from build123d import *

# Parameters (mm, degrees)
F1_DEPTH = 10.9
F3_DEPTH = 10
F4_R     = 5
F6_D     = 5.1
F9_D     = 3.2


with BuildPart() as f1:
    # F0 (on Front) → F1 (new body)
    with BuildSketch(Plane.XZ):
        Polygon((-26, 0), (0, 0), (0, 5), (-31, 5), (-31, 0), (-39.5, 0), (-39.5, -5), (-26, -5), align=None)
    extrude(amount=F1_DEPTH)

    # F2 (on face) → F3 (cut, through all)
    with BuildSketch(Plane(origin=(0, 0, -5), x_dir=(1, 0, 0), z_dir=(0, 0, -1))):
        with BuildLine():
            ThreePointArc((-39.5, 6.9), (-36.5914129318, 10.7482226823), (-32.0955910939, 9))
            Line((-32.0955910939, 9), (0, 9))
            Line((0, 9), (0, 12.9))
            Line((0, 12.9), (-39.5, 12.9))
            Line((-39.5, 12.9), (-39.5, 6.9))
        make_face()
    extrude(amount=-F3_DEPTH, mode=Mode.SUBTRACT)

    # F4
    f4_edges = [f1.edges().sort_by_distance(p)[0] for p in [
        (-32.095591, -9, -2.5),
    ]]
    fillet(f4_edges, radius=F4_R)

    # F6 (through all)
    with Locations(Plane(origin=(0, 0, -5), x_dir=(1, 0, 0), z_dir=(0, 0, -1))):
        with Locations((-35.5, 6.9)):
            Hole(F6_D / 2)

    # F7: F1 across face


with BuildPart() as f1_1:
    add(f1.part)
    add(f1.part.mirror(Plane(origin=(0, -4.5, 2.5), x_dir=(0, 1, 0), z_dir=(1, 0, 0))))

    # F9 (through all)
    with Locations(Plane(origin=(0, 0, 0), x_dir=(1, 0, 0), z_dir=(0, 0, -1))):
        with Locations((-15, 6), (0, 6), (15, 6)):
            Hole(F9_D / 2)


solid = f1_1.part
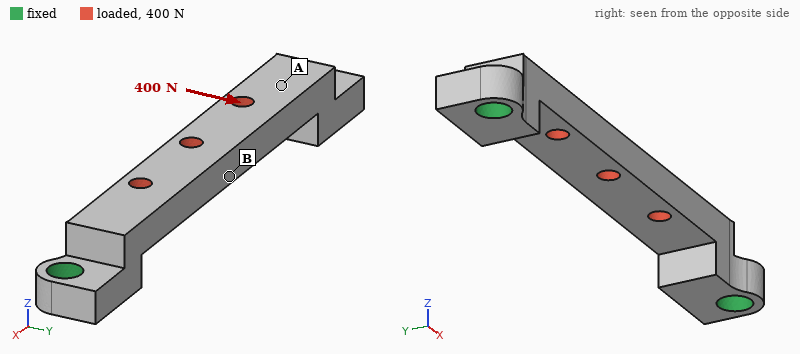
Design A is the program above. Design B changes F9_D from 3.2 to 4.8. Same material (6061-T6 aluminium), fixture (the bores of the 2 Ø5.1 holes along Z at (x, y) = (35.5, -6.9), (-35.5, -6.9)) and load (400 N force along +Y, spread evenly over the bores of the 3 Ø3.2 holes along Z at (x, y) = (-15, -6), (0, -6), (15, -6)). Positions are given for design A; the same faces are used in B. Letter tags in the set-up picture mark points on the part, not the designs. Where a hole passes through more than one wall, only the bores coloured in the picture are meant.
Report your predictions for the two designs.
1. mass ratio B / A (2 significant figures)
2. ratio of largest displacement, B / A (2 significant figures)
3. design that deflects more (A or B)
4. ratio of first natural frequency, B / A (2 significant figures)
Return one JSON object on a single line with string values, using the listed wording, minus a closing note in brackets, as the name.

{"mass ratio B / A": "0.96", "ratio of largest displacement, B / A": "1.1", "design that deflects more": "B", "ratio of first natural frequency, B / A": "0.98"}
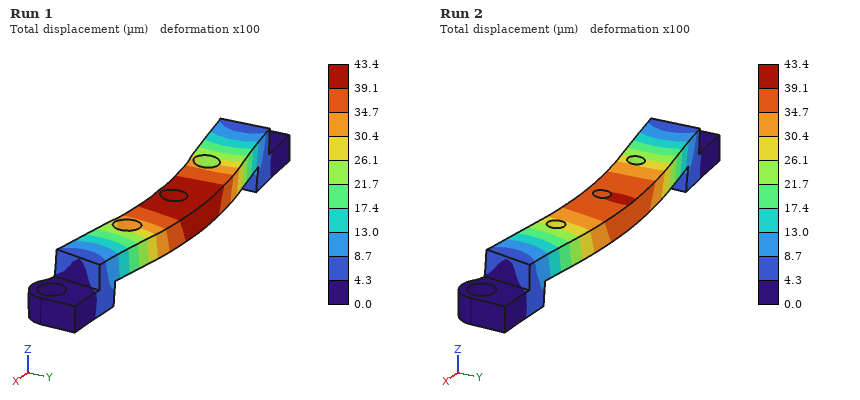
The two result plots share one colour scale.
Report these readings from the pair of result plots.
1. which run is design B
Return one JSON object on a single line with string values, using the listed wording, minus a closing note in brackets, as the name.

{"which run is design B": "Run 1"}
